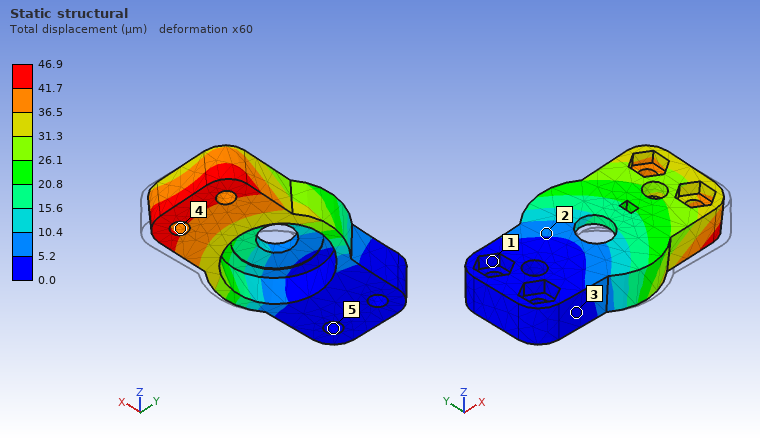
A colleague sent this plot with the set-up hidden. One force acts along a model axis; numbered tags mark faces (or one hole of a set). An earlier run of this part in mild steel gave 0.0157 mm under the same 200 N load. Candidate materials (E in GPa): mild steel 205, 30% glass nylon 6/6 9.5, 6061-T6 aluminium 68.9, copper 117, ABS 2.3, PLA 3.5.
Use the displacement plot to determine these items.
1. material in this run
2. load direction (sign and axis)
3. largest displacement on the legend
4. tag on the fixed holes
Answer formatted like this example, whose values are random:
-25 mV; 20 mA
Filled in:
6061-T6 aluminium; +Y; 46.9 µm; 5
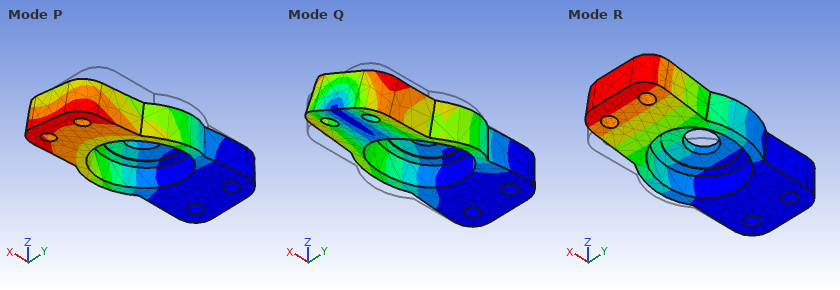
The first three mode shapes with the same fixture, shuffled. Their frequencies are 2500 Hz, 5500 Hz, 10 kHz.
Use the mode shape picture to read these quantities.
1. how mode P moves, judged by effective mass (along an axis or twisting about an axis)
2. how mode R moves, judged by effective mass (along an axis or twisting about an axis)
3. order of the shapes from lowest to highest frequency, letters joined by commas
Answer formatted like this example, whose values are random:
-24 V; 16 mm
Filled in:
along Y; along Z; R, P, Q
